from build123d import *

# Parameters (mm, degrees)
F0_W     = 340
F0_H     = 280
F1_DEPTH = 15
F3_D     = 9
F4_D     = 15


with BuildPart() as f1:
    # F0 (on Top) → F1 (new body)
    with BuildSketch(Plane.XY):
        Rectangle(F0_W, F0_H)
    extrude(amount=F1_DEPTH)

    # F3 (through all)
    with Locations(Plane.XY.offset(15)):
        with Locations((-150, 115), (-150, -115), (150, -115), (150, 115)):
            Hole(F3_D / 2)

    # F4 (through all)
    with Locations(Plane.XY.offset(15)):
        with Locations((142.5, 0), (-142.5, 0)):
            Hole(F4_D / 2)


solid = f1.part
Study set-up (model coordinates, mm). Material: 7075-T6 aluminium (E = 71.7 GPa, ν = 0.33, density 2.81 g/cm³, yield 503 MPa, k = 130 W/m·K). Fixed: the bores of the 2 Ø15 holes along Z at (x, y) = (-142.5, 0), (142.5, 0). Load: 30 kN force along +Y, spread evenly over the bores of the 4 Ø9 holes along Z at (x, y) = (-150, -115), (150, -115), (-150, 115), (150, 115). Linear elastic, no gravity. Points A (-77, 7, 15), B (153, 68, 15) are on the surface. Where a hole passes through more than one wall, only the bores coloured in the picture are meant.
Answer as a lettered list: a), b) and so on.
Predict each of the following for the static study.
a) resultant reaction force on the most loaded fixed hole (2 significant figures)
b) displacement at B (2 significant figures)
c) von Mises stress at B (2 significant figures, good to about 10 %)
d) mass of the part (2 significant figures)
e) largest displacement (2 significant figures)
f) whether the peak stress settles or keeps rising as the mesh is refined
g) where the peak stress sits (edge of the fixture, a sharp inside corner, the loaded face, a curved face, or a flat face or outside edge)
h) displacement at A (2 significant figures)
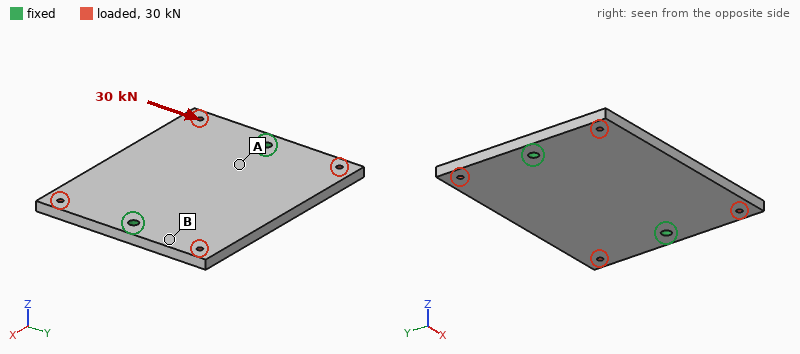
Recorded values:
a) 15 kN
b) 10 µm
c) 9.8 MPa
d) 4.0 kg
e) 20 µm
f) keeps rising
g) edge of the fixture
h) 7.4 µm
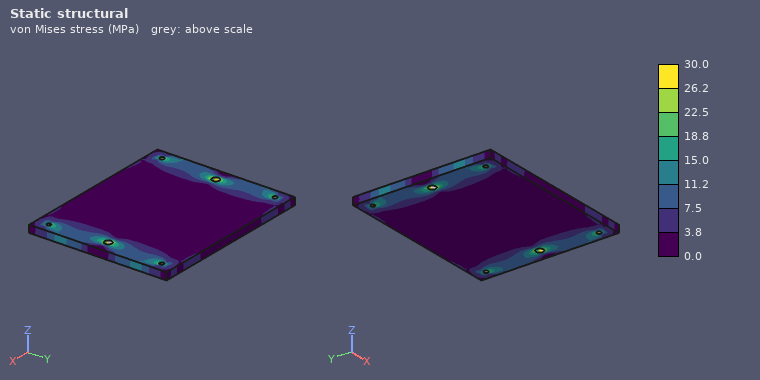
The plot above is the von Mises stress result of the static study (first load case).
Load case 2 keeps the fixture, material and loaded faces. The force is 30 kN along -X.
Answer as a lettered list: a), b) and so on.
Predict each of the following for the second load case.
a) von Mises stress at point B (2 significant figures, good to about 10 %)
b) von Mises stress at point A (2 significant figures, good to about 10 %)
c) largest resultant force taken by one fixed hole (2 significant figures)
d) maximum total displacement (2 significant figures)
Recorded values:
a) 3.3 MPa
b) 7.2 MPa
c) 15 kN
d) 36 µm
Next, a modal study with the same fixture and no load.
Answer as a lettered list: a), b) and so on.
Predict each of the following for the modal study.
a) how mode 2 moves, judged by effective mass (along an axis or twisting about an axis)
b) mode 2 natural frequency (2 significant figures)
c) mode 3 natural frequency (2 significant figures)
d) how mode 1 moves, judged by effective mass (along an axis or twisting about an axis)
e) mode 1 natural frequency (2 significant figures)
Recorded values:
a) along Z
b) 520 Hz
c) 800 Hz
d) twisting about X
e) 370 Hz
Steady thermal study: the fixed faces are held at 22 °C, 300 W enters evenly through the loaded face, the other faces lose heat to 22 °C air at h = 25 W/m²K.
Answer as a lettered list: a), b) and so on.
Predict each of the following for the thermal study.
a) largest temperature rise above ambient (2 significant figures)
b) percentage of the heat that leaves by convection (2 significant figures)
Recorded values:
a) 53 K
b) 39 %
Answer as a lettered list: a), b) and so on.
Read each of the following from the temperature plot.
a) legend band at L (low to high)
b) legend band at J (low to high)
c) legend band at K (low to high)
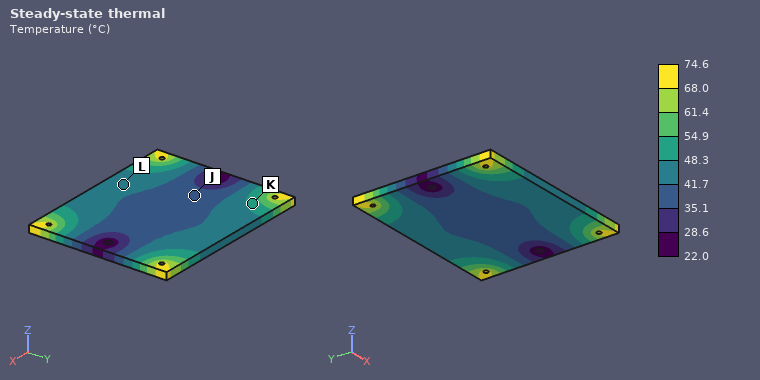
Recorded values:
a) 41.7 to 48.3 °C
b) 35.1 to 41.7 °C
c) 48.3 to 54.9 °C
